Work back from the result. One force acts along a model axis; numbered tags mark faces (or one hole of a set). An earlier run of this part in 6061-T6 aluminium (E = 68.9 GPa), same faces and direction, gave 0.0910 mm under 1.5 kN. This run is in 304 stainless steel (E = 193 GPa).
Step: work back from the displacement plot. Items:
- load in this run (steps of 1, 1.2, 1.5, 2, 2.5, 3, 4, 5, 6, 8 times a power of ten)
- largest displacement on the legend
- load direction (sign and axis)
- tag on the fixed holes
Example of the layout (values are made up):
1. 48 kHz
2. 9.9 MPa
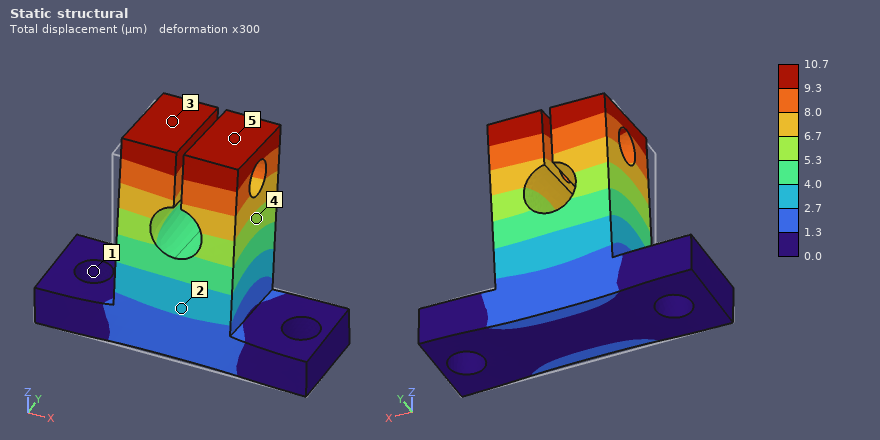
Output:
1. 500 N
2. 10.7 µm
3. +Y
4. 1
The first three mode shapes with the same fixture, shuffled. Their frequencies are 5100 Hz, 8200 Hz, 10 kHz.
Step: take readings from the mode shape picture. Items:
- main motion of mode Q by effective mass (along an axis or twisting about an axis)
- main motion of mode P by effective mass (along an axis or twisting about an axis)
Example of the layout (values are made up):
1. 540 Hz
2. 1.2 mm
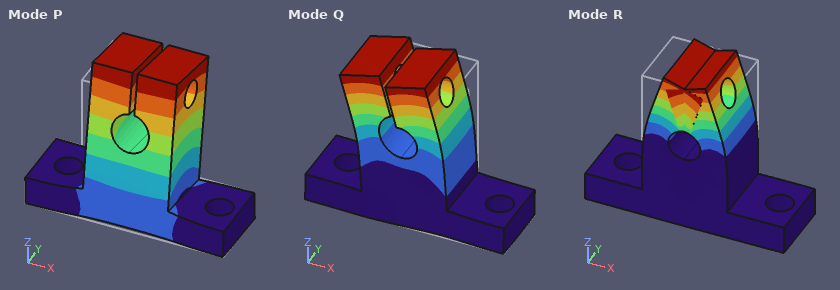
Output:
1. along X
2. along Y
